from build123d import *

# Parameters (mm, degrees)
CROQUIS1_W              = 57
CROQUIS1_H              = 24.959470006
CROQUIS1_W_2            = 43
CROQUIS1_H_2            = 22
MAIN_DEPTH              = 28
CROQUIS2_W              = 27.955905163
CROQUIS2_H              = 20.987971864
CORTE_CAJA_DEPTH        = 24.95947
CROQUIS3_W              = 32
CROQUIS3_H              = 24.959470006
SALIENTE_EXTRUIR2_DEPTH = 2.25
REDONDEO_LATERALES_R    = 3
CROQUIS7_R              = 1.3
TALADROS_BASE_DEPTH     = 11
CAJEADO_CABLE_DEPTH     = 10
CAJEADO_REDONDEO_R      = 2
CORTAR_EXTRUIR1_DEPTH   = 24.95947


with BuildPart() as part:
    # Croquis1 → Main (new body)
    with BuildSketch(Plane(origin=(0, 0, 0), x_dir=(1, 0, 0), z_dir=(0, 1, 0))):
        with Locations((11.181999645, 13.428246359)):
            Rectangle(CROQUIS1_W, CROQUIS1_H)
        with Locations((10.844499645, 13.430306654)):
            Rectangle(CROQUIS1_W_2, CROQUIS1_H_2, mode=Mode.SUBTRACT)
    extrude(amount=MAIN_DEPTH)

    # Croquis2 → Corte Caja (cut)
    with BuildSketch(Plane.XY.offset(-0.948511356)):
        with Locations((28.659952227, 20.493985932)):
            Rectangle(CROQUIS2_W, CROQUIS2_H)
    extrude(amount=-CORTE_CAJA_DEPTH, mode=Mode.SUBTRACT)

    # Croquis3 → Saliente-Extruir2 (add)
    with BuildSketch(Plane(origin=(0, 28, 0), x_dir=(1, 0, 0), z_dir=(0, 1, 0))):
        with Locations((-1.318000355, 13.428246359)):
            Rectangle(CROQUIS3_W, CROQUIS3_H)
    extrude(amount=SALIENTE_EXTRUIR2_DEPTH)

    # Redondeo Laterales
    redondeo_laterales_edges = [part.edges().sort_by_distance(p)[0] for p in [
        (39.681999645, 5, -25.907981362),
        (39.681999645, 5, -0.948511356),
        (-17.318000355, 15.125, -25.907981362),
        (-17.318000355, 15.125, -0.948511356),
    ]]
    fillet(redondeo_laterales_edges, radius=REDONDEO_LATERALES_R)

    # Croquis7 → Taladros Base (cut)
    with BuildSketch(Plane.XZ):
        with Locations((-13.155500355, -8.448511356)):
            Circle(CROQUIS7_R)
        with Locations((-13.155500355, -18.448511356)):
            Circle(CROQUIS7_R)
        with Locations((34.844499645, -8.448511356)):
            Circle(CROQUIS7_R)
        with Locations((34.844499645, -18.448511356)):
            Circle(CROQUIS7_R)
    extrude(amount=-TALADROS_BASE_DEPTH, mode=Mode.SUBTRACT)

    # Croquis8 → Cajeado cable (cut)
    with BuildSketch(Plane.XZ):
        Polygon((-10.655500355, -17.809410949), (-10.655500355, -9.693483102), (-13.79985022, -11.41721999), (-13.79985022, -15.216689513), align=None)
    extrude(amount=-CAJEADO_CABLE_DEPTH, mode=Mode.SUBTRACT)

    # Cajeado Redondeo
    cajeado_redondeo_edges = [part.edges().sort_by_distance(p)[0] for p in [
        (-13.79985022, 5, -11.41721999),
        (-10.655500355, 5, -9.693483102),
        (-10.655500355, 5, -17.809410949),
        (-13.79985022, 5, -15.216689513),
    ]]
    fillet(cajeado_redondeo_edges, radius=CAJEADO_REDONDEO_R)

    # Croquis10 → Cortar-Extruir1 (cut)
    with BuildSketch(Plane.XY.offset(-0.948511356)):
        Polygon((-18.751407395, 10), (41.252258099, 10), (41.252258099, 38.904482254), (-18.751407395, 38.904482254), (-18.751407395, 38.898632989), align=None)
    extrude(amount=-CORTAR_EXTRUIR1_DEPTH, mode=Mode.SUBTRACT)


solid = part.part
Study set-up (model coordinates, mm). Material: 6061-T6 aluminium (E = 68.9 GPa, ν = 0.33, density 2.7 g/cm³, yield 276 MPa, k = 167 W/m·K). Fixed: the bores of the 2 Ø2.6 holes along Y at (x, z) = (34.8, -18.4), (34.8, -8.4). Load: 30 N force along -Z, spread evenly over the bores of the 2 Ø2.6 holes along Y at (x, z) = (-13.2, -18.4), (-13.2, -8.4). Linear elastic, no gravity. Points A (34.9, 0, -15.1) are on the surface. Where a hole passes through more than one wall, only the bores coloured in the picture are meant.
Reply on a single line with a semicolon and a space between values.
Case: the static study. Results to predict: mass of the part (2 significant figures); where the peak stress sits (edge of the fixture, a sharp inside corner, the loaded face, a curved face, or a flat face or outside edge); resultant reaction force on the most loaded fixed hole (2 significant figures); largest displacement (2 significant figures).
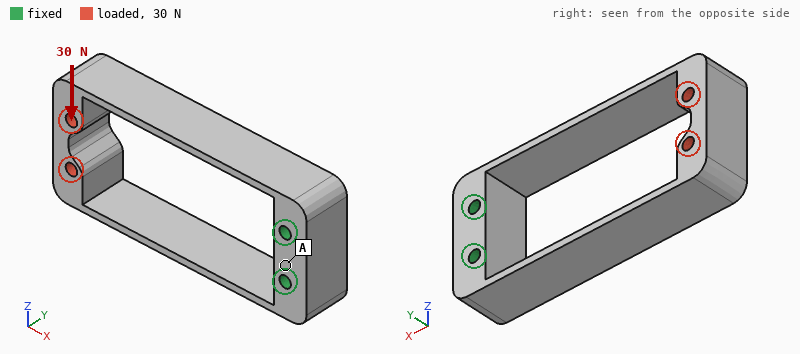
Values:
12 g; a flat face or outside edge; 83 N; 0.59 mm
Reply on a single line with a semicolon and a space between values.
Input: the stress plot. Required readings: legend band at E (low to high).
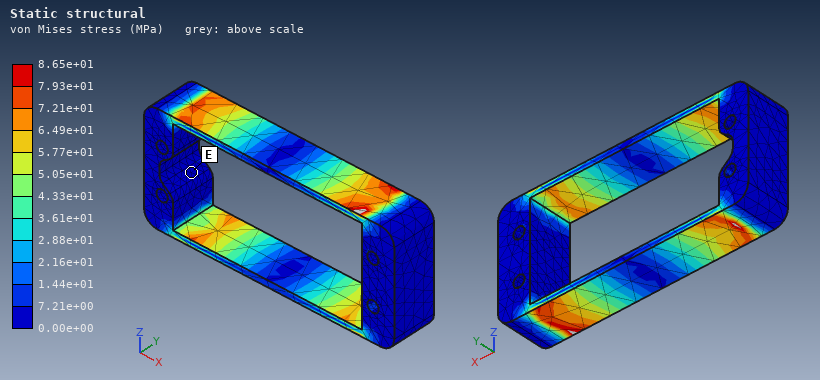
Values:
0.00e+00 to 7.21e+00 MPa
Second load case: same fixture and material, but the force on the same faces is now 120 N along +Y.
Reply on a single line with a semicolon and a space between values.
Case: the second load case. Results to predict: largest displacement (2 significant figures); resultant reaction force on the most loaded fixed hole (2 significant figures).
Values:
0.36 mm; 60 N
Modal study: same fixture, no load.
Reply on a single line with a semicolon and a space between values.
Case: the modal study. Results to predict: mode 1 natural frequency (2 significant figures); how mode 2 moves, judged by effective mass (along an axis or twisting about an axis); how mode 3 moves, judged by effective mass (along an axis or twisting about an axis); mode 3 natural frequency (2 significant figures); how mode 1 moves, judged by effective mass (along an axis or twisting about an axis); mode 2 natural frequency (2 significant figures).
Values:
520 Hz; along Y; twisting about X; 3000 Hz; along Z; 1400 Hz
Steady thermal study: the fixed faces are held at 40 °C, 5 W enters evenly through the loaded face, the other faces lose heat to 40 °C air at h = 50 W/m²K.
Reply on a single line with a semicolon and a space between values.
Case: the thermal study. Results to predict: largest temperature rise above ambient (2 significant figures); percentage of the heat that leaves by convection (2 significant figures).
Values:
29 K; 51 %
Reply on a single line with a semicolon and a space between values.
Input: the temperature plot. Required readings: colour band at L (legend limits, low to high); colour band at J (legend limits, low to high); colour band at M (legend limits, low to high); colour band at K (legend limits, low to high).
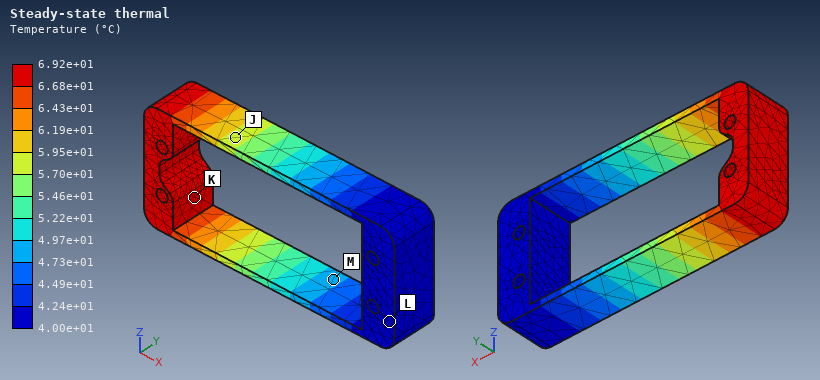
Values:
4.00e+01 to 4.24e+01 °C; 5.70e+01 to 5.95e+01 °C; 4.73e+01 to 4.97e+01 °C; 6.68e+01 to 6.92e+01 °C
